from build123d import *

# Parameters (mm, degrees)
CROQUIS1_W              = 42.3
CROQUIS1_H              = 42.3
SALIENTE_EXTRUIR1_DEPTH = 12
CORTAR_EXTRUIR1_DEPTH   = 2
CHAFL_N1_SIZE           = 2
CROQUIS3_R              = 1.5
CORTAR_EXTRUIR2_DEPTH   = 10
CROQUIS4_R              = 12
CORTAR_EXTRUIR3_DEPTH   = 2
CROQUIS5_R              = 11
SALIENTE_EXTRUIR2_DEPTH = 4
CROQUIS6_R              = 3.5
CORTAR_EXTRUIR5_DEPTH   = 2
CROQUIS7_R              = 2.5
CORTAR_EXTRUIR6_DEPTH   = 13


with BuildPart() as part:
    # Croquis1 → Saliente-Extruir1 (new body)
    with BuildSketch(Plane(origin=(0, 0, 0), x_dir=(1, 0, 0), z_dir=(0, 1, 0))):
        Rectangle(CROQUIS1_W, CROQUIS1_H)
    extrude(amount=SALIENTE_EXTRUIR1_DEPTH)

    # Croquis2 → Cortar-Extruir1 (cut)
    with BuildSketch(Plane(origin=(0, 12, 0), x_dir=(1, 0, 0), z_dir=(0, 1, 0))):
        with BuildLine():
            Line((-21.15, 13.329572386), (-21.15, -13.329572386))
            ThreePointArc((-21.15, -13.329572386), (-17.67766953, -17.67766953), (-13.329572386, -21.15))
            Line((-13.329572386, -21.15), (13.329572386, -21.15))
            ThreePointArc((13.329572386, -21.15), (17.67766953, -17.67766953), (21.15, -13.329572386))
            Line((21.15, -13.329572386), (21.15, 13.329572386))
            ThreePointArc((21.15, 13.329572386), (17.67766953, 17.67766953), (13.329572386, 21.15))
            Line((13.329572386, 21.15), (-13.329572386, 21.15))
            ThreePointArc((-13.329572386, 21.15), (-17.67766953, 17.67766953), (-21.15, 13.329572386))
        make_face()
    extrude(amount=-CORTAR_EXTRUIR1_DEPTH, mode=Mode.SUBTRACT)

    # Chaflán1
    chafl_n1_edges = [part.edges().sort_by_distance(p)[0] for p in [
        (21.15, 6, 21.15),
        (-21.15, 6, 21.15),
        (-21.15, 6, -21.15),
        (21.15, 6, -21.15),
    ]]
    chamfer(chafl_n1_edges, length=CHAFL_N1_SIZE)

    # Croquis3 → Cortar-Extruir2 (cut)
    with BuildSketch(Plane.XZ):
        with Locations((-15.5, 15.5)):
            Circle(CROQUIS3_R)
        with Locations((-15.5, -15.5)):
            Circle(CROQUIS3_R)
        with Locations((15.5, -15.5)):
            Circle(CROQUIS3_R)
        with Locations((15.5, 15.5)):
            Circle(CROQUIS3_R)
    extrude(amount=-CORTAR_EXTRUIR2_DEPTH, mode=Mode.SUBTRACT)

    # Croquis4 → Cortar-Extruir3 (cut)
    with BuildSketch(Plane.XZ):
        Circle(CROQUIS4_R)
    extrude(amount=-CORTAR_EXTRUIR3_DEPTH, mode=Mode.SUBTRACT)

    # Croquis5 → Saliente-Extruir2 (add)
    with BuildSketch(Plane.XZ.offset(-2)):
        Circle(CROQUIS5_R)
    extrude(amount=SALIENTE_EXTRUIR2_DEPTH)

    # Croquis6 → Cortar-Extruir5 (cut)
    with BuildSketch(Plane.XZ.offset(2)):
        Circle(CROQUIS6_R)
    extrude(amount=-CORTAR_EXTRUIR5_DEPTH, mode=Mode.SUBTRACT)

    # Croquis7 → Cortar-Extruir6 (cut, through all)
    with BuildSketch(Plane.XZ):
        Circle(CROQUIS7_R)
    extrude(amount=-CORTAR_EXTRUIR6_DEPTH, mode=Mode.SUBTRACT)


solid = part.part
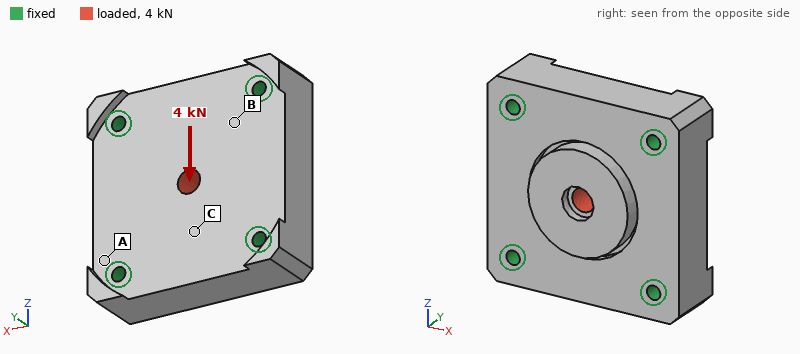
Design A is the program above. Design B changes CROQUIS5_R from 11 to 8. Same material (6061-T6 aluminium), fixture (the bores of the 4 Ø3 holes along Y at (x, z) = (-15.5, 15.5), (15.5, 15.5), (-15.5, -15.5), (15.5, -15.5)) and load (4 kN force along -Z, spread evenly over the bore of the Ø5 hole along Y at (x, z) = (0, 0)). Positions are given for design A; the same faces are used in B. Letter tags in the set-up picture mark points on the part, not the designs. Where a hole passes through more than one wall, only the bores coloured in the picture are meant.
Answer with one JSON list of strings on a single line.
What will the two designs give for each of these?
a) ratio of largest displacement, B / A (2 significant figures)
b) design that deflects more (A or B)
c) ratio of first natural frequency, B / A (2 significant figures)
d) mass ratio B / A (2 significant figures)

["1.1", "B", "1.0", "0.96"]
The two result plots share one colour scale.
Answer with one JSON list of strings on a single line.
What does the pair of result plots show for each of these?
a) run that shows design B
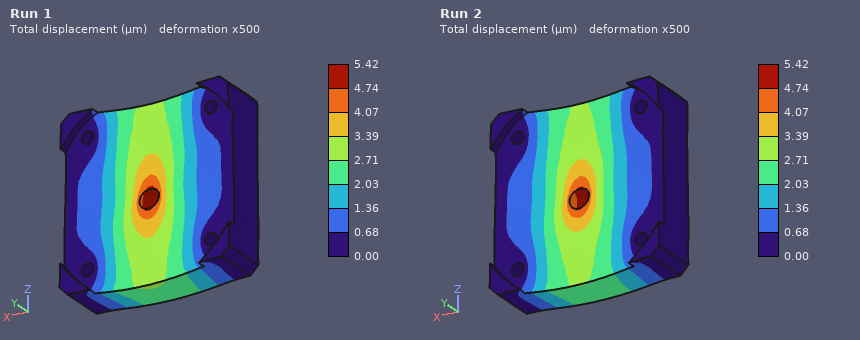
["Run 1"]
